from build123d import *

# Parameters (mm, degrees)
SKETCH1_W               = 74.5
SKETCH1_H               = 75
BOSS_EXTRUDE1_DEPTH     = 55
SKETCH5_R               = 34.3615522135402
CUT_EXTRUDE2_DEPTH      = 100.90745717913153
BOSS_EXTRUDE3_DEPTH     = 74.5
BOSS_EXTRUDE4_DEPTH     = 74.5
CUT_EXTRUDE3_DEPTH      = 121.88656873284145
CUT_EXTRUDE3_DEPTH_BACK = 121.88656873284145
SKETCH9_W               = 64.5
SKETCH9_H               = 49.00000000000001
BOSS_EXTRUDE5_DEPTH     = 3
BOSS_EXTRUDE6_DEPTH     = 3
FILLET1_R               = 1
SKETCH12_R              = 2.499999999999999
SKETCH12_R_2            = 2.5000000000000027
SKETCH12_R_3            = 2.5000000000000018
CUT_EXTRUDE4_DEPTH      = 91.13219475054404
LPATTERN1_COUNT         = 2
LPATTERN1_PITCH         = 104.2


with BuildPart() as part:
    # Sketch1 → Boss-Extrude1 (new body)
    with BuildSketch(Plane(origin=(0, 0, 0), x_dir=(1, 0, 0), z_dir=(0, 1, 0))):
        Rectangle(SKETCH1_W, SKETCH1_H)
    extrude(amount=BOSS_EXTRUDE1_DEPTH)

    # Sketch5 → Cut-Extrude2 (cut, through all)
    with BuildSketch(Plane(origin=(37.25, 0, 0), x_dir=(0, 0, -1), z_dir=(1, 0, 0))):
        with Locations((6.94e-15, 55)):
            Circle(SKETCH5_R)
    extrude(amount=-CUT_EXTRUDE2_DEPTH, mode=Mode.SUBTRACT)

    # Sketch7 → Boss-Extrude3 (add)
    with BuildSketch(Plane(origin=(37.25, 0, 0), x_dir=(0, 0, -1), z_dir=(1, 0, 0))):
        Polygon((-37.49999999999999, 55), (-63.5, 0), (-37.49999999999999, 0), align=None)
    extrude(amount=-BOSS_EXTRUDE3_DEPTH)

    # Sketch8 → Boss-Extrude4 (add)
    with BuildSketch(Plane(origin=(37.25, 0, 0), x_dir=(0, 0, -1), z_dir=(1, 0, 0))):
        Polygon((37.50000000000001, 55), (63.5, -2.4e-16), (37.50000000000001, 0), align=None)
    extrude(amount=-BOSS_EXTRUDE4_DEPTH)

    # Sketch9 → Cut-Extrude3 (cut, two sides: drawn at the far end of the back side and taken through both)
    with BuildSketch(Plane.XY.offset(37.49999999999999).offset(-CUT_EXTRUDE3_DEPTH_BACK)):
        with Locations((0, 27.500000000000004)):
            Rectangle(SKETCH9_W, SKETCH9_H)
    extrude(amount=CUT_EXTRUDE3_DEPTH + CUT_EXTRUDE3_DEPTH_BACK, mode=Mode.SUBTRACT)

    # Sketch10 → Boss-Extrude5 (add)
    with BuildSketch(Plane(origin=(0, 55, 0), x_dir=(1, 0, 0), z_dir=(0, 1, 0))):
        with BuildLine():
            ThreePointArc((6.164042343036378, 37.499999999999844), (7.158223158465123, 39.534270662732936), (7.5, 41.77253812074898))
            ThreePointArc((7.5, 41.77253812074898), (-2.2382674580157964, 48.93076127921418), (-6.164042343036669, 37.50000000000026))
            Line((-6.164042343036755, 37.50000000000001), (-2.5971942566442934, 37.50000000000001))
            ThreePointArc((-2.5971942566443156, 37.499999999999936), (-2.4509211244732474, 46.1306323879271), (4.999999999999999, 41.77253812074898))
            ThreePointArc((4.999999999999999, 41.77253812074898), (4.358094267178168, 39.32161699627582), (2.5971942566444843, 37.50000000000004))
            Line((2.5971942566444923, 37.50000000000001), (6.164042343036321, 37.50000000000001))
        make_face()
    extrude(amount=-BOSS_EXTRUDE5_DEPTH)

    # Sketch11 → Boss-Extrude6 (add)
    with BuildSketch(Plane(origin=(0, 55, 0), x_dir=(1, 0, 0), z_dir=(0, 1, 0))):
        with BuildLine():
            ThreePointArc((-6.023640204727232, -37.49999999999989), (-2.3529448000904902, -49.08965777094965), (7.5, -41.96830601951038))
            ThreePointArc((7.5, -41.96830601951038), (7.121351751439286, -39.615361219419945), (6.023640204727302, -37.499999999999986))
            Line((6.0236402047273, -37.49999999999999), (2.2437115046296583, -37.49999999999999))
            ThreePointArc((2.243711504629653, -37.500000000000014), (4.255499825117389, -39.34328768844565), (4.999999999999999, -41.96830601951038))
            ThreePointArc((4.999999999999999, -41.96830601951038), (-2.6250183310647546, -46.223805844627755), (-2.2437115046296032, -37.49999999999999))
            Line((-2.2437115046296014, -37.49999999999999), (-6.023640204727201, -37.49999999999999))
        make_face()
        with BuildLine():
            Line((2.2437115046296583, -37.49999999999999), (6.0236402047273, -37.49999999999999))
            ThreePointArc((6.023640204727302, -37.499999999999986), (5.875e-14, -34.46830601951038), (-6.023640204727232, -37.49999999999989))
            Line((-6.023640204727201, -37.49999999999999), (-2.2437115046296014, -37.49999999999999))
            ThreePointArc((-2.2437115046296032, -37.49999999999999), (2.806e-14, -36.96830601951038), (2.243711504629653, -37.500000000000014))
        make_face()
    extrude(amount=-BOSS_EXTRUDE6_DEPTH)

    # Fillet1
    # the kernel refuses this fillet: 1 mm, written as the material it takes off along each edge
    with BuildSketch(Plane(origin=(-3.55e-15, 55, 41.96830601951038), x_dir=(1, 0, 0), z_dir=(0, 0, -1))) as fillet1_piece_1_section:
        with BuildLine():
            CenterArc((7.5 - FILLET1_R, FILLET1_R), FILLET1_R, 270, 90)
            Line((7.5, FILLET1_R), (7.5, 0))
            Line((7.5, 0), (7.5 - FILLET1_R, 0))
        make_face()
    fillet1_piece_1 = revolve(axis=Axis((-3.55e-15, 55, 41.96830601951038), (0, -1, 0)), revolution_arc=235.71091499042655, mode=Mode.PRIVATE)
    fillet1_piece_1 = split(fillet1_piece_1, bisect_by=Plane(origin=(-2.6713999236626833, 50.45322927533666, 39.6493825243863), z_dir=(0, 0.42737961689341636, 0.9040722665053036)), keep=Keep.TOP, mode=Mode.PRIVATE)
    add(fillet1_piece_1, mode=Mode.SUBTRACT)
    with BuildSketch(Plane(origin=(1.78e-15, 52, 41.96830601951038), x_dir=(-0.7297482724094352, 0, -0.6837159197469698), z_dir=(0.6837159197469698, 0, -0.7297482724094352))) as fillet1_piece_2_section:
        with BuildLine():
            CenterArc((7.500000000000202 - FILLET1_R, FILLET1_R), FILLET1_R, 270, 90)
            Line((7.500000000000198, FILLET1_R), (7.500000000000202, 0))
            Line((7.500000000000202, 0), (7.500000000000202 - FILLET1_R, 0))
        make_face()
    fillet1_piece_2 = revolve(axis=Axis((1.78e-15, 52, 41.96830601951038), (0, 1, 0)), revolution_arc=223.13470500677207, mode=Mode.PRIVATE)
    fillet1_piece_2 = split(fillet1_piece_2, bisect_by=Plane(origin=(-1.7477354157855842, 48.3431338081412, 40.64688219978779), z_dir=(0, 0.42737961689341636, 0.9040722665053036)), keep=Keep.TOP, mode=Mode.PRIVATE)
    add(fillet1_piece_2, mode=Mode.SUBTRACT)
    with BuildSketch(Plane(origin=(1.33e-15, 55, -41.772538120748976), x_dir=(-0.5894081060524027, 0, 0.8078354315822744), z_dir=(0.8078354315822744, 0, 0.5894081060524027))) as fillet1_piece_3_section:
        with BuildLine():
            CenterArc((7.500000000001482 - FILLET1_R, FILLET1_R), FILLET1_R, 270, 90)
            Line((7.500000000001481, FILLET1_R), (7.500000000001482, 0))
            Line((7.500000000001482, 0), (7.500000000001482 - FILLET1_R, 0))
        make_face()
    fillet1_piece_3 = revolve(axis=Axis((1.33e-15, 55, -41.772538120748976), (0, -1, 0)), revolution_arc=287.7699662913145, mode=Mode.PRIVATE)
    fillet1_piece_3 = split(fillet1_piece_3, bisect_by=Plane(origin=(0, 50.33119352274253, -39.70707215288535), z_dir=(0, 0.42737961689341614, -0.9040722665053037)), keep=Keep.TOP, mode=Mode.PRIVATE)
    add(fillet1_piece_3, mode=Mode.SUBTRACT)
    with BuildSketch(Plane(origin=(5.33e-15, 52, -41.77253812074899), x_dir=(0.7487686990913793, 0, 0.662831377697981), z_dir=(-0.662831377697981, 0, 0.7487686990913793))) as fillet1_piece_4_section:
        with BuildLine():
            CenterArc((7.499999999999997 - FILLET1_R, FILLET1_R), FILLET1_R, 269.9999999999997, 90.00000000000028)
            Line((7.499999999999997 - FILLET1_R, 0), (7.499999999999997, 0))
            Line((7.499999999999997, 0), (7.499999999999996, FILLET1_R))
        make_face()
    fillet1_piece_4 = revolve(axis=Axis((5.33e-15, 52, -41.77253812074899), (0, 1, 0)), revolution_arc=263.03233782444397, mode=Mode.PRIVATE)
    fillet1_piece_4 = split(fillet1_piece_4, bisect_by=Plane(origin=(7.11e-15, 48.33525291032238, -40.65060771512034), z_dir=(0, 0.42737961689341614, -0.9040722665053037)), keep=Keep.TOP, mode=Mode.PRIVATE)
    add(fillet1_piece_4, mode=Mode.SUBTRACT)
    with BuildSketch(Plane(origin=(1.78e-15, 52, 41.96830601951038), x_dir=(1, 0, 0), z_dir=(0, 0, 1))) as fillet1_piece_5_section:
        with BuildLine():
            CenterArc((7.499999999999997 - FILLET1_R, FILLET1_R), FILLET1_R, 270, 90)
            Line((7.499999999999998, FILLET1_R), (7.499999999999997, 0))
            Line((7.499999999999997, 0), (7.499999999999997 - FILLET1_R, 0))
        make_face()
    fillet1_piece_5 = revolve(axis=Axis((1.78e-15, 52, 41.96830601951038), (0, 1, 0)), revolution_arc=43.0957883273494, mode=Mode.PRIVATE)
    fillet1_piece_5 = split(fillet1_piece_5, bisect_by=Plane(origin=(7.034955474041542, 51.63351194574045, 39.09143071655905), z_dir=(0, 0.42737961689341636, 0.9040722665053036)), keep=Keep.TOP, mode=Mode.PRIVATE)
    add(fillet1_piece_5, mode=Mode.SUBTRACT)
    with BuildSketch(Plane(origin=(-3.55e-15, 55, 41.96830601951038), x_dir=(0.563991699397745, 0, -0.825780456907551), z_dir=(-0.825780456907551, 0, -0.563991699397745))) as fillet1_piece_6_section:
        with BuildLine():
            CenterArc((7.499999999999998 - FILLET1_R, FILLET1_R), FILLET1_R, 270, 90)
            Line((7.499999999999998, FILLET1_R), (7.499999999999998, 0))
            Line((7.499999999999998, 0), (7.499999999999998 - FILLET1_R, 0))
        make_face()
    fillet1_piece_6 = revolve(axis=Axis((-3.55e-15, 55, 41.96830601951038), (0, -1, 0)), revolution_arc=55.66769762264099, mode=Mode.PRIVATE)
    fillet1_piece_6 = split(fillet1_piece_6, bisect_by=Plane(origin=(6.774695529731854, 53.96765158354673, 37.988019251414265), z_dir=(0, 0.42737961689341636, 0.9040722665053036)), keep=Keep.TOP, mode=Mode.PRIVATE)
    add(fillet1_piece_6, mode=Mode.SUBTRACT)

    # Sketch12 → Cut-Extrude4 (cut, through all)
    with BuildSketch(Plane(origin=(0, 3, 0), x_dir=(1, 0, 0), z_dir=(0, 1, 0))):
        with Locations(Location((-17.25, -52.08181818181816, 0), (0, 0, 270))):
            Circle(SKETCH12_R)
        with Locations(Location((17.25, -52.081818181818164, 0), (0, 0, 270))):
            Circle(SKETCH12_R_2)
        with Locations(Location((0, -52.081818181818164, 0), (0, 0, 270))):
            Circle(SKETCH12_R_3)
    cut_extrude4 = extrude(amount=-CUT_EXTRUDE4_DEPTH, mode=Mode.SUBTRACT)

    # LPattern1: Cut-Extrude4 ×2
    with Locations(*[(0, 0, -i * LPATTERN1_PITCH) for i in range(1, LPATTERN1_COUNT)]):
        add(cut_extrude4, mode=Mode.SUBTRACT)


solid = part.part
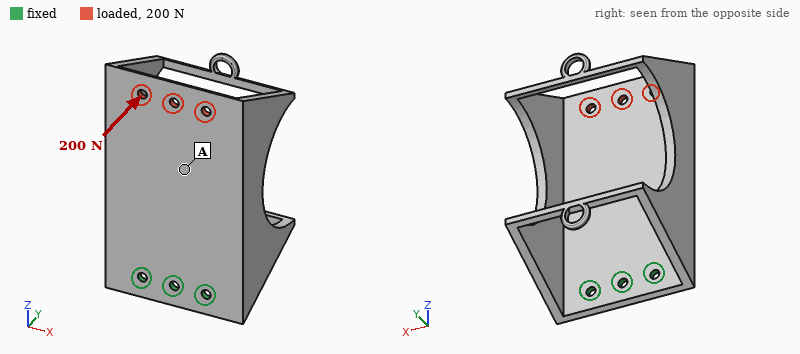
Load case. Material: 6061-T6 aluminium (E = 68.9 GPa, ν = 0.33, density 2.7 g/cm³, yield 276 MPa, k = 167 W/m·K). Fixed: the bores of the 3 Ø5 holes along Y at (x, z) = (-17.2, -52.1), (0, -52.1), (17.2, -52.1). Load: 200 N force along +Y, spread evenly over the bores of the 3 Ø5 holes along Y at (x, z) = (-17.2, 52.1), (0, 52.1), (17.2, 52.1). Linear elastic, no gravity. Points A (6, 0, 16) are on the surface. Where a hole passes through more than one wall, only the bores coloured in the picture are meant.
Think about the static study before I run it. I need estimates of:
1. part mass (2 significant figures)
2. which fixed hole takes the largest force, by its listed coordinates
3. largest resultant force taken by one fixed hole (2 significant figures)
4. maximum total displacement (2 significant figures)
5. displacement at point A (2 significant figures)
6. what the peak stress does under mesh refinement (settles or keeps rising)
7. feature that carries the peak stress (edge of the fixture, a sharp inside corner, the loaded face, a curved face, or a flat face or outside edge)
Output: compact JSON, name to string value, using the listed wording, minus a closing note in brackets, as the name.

{"part mass": "170 g", "which fixed hole takes the largest force, by its listed coordinates": "(0, -52.1)", "largest resultant force taken by one fixed hole": "200 N", "maximum total displacement": "1.7 mm", "displacement at point A": "0.91 mm", "what the peak stress does under mesh refinement": "keeps rising", "feature that carries the peak stress": "edge of the fixture"}
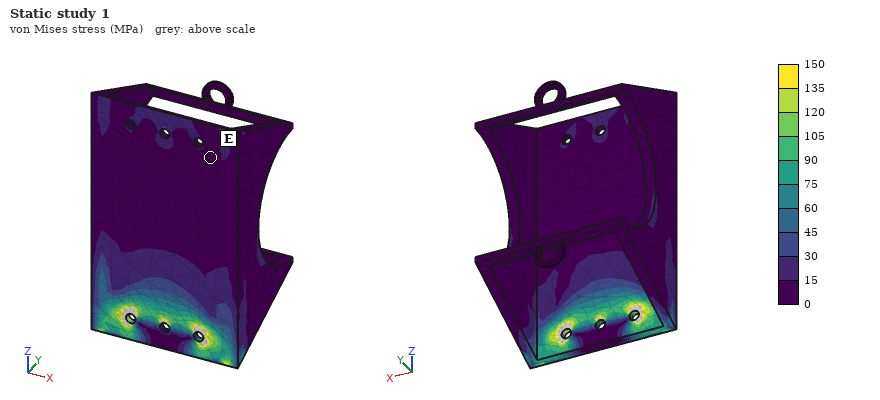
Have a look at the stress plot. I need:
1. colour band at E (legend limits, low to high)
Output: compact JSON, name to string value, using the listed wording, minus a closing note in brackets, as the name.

{"colour band at E": "0 to 15 MPa"}
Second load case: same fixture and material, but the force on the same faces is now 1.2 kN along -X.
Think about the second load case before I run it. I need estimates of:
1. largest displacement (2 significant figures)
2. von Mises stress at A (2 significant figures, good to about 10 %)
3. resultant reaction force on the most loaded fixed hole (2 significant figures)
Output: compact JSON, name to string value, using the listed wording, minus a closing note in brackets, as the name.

{"largest displacement": "0.16 mm", "von Mises stress at A": "11 MPa", "resultant reaction force on the most loaded fixed hole": "3.3 kN"}
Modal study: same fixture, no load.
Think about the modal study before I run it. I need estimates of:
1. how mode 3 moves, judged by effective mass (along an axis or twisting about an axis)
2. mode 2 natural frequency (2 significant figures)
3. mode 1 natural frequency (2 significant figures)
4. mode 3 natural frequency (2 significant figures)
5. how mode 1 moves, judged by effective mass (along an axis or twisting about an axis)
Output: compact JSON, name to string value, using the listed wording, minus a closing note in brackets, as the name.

{"how mode 3 moves, judged by effective mass": "along X", "mode 2 natural frequency": "400 Hz", "mode 1 natural frequency": "230 Hz", "mode 3 natural frequency": "1200 Hz", "how mode 1 moves, judged by effective mass": "along Y"}
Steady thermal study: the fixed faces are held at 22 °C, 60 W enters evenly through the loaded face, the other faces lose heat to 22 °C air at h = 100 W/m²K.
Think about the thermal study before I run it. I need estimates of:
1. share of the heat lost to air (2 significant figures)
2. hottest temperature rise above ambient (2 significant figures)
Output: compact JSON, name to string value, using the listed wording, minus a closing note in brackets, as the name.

{"share of the heat lost to air": "85 %", "hottest temperature rise above ambient": "58 K"}
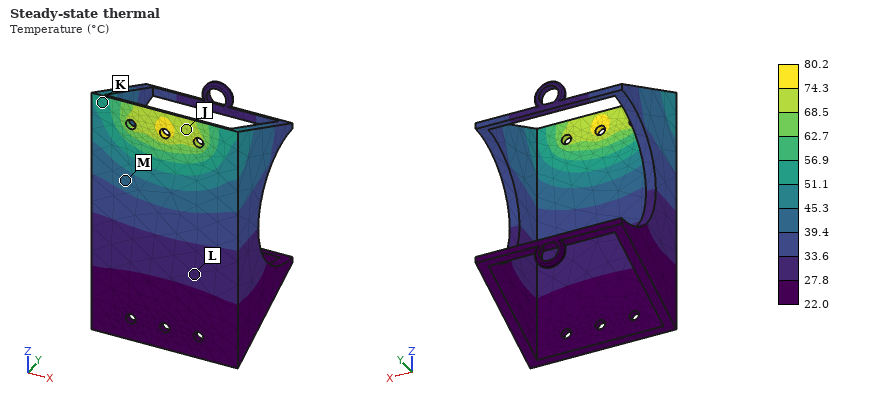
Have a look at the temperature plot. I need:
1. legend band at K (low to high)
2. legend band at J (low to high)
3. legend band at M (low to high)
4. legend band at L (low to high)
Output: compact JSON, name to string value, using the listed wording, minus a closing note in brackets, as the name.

{"legend band at K": "51.1 to 56.9 °C", "legend band at J": "68.5 to 74.3 °C", "legend band at M": "39.4 to 45.3 °C", "legend band at L": "27.8 to 33.6 °C"}
